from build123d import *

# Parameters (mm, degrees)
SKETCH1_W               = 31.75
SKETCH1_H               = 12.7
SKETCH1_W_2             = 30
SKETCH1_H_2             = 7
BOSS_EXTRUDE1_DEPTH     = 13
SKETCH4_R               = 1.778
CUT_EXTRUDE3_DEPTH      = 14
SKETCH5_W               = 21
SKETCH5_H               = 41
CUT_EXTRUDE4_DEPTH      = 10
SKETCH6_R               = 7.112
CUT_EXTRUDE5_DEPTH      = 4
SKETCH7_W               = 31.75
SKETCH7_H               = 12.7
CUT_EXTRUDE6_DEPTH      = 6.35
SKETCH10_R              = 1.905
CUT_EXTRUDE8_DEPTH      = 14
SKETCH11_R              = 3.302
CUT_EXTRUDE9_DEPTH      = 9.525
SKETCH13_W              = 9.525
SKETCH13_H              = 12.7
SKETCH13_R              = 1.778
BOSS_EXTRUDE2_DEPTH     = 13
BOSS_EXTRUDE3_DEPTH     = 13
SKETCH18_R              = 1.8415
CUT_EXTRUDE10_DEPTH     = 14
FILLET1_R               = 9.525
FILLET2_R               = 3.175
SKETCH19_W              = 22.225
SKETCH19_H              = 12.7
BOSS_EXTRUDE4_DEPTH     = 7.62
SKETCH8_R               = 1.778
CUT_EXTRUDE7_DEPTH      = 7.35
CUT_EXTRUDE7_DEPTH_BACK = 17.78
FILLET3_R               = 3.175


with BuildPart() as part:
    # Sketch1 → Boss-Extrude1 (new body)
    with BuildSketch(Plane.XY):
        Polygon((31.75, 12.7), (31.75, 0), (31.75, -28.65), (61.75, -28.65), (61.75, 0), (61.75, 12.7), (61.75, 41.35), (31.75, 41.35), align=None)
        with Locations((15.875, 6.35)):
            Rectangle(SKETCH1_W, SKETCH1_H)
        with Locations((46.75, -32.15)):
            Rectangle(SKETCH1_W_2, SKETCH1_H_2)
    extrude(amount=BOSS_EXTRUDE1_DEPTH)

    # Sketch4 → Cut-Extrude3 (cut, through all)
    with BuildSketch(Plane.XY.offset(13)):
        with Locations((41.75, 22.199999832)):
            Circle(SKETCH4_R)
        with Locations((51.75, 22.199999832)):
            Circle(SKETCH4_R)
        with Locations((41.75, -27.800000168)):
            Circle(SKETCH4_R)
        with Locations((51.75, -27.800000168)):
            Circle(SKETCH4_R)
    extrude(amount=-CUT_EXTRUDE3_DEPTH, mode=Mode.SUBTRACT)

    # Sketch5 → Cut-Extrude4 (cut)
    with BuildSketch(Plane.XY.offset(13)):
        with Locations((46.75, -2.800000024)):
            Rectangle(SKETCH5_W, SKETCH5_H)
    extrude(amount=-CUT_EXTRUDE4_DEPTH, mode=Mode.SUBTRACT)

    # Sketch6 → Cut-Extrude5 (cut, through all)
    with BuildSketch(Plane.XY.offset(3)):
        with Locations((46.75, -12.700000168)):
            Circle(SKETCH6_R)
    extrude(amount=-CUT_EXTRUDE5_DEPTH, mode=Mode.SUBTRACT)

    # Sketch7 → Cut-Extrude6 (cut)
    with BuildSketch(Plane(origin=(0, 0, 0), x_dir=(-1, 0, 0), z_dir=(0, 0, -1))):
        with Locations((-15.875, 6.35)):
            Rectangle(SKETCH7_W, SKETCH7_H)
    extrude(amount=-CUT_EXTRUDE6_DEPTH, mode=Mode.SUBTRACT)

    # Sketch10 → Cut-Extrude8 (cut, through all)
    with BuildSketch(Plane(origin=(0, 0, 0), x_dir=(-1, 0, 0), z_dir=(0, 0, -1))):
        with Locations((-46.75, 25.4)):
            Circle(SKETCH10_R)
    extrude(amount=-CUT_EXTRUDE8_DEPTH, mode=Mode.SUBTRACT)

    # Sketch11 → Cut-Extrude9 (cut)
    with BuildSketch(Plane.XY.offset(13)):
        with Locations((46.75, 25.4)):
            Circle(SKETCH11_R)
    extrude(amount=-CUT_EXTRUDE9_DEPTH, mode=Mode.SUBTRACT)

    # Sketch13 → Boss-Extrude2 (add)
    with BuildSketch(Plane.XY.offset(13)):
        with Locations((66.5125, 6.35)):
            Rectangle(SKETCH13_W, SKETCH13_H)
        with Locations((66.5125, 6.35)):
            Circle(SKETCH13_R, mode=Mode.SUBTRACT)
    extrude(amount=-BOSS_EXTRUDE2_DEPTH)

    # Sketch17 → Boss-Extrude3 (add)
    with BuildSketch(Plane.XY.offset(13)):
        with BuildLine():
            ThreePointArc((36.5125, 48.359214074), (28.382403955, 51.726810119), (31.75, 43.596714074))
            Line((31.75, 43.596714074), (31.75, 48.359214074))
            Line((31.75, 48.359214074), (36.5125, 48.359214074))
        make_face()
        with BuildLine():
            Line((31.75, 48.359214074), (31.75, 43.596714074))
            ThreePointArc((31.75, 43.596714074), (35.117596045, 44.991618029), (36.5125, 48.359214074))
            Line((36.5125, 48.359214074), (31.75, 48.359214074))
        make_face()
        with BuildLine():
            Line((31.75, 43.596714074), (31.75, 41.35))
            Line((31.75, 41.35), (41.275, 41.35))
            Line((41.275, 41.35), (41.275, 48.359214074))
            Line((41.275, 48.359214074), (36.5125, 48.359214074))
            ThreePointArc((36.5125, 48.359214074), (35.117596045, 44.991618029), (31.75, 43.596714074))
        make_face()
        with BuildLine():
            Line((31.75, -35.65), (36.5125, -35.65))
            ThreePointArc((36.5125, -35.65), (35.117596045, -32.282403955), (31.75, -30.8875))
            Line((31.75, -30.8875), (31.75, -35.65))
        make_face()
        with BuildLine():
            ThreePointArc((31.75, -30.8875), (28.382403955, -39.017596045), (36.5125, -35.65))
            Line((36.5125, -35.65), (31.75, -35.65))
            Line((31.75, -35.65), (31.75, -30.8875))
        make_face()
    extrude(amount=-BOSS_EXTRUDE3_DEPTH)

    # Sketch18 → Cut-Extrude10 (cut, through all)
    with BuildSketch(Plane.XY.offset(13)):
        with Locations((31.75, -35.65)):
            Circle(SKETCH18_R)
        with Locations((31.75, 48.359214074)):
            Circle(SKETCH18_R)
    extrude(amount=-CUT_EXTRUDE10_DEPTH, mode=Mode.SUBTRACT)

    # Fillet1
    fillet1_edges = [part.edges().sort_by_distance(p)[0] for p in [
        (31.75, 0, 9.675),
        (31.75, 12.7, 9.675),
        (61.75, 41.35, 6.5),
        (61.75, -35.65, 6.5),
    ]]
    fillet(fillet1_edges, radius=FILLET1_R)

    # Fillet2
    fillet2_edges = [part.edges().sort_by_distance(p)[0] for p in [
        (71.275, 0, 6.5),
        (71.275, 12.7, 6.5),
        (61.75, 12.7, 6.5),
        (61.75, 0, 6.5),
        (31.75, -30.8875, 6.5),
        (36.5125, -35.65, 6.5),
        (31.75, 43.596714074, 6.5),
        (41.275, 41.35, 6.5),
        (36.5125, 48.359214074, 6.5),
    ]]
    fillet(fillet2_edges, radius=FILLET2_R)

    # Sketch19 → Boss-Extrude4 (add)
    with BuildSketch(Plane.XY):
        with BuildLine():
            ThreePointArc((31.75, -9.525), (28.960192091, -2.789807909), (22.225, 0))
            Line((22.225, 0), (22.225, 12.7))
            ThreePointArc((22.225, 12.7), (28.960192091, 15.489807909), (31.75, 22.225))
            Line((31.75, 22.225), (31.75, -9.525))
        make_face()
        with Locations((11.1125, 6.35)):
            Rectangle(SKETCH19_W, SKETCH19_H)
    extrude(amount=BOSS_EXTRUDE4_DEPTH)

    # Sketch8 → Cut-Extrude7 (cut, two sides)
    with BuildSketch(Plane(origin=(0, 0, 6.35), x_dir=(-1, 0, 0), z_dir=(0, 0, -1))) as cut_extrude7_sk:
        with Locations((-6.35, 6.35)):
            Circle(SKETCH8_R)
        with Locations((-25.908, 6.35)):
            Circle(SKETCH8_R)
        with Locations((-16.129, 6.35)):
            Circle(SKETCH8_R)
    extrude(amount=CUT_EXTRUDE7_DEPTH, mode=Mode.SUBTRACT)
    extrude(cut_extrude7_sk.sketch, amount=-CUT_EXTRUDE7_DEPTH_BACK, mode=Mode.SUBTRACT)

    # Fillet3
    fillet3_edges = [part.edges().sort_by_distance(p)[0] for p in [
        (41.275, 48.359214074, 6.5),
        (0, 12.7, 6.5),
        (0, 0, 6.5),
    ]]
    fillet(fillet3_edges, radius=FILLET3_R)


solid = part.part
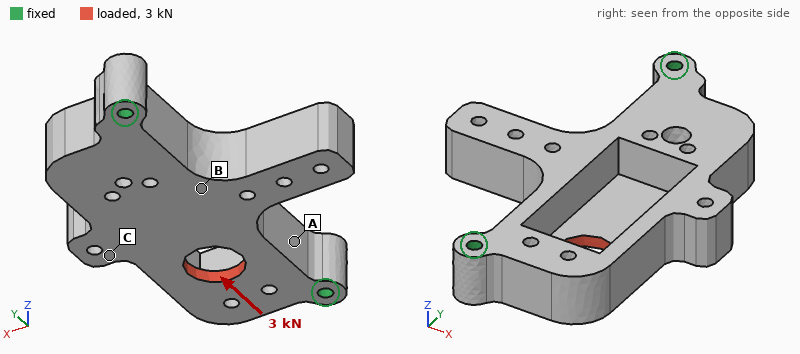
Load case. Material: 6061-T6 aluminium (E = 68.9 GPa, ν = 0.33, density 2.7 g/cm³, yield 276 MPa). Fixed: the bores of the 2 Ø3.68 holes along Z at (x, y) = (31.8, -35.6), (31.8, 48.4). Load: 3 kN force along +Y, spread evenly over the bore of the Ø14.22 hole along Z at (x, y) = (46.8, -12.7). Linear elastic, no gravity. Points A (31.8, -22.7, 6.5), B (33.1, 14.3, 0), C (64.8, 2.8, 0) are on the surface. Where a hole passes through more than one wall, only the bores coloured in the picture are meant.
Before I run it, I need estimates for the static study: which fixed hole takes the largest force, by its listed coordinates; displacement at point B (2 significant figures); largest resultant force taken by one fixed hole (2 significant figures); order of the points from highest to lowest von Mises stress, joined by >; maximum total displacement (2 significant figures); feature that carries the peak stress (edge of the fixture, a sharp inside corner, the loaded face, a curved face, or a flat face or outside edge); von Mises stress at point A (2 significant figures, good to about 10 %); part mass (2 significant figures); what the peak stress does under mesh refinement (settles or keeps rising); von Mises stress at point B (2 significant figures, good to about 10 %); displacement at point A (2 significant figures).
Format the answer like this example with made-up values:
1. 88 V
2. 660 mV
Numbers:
1. (31.8, -35.6)
2. 8.3 µm
3. 1.7 kN
4. A > B > C
5. 18 µm
6. edge of the fixture
7. 24 MPa
8. 77 g
9. keeps rising
10. 9.8 MPa
11. 4.9 µm
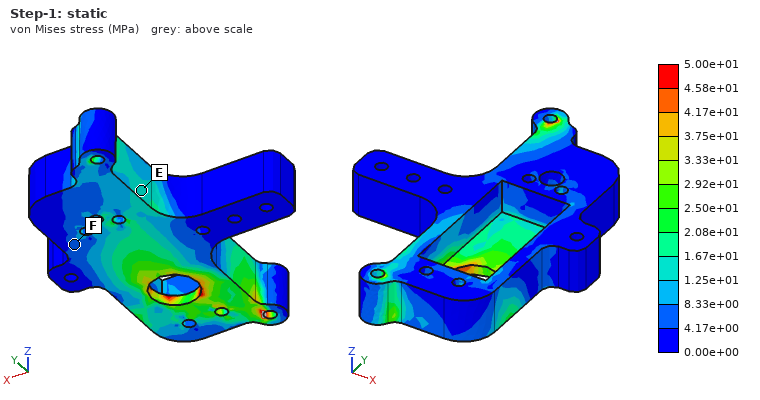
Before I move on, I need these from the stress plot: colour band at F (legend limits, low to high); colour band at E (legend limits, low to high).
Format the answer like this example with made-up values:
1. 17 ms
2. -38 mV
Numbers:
1. 4.17e+00 to 8.33e+00 MPa
2. 1.25e+01 to 1.67e+01 MPa
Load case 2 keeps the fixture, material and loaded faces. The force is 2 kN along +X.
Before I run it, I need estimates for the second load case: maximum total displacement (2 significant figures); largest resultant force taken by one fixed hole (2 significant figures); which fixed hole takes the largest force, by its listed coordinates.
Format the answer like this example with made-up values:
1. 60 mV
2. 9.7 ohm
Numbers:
1. 39 µm
2. 1.6 kN
3. (31.8, -35.6)
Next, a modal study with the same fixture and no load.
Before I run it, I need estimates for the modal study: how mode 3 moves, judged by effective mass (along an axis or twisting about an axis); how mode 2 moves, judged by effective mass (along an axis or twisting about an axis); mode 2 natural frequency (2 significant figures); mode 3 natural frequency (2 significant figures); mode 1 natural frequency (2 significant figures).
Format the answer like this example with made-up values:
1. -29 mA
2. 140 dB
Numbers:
1. along X
2. along Z
3. 4100 Hz
4. 6800 Hz
5. 2800 Hz
